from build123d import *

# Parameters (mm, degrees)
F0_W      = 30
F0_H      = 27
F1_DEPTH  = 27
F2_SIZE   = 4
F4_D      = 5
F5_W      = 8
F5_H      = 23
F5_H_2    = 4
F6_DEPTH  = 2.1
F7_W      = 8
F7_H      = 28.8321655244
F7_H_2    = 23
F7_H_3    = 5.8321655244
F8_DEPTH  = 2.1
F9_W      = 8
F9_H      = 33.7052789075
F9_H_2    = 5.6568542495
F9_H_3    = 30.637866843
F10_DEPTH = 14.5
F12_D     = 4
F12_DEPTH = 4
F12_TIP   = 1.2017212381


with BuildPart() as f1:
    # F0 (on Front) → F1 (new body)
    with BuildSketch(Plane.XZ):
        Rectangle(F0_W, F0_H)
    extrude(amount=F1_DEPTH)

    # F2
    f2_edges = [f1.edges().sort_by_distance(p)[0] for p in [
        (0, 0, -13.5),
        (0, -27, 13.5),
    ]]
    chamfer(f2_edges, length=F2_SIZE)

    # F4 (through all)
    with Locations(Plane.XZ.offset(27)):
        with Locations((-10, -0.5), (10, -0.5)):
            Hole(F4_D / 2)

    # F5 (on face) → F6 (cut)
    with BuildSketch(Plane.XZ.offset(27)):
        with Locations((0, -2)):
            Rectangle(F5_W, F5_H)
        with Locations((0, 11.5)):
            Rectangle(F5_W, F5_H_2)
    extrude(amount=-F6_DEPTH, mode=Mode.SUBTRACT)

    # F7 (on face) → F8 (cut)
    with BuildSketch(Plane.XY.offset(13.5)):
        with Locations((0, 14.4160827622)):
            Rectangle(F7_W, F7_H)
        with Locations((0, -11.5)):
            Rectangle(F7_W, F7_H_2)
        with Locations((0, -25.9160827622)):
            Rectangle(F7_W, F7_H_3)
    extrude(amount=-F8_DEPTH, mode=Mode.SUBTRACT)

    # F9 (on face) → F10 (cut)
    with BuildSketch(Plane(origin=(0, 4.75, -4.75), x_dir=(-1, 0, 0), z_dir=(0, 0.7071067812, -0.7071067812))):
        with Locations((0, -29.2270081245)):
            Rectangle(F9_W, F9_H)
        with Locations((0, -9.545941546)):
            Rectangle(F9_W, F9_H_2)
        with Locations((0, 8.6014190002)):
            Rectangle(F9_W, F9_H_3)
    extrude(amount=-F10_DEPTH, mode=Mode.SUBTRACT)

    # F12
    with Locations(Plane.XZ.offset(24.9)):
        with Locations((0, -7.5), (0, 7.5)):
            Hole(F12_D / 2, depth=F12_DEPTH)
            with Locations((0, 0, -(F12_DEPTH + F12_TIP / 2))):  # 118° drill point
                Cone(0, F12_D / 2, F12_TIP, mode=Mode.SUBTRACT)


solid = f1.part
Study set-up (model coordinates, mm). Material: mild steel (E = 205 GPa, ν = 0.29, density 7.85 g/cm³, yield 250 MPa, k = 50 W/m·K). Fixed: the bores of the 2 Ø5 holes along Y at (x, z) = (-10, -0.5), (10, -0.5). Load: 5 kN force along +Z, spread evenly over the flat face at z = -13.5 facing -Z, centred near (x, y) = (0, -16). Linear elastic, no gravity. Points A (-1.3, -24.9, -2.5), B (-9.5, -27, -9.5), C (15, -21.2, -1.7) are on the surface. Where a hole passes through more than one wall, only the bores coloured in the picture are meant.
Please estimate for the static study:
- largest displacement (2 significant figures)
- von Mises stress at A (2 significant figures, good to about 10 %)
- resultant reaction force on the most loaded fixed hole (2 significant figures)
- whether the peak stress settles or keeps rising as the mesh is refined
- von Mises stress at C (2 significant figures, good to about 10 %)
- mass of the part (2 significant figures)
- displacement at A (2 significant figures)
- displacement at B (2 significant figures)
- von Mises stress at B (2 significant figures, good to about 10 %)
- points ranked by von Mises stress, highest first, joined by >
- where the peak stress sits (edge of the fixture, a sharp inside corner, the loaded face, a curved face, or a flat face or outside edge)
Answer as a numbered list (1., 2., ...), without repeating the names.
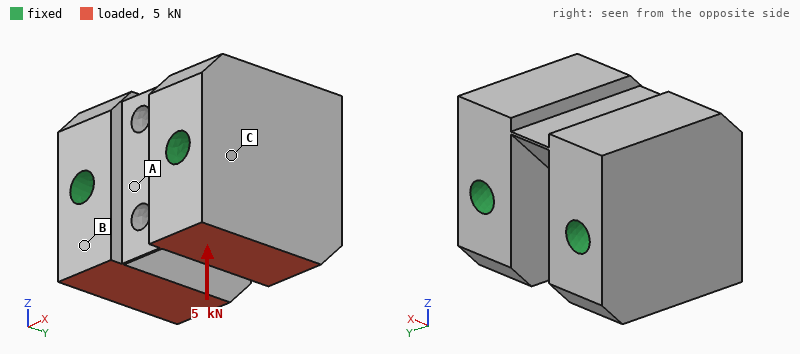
1. 0.72 µm
2. 2.4 MPa
3. 2.5 kN
4. keeps rising
5. 5.6 MPa
6. 130 g
7. 0.21 µm
8. 0.48 µm
9. 11 MPa
10. B > C > A
11. edge of the fixture
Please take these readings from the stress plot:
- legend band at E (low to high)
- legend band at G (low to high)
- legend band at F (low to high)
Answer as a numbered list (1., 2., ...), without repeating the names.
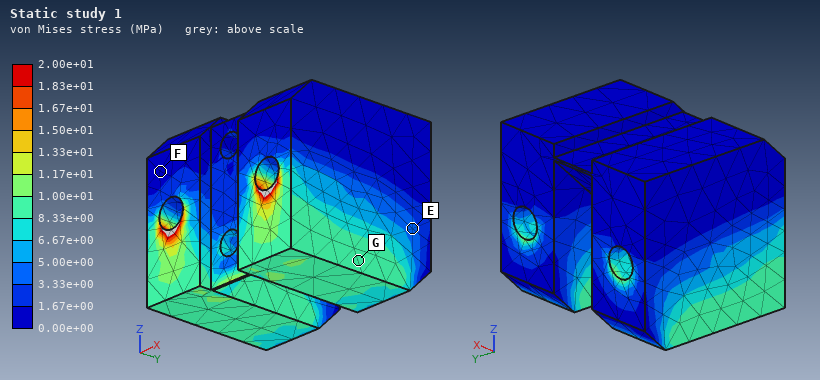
1. 3.33e+00 to 5.00e+00 MPa
2. 8.33e+00 to 1.00e+01 MPa
3. 0.00e+00 to 1.67e+00 MPa
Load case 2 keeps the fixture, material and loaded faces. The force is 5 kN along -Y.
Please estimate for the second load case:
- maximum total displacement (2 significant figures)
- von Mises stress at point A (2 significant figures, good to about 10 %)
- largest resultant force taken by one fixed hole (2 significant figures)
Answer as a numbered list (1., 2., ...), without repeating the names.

1. 2.7 µm
2. 6.1 MPa
3. 2.5 kN
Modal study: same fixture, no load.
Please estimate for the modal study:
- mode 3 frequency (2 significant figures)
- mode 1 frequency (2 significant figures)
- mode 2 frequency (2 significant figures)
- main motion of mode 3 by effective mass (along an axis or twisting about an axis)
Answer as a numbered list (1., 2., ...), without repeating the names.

1. 48 kHz
2. 43 kHz
3. 44 kHz
4. along X
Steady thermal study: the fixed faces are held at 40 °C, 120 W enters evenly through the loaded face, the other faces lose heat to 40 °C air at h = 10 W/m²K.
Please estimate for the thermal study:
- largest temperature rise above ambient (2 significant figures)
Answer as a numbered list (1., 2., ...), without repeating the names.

1. 51 K
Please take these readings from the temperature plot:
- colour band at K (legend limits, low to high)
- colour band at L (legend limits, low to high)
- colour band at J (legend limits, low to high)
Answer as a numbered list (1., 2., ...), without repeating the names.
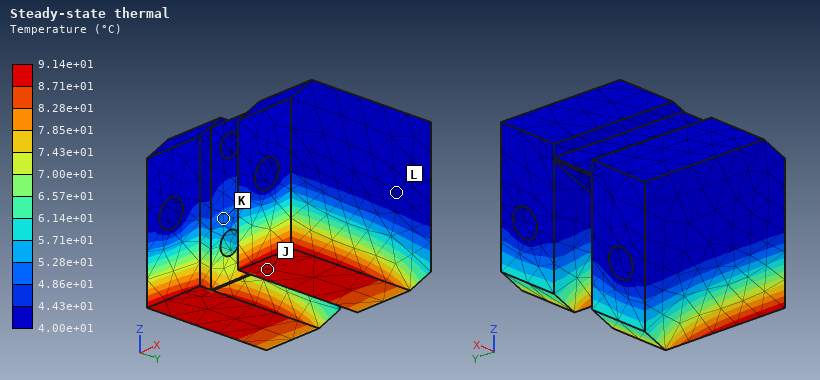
1. 4.86e+01 to 5.28e+01 °C
2. 4.00e+01 to 4.43e+01 °C
3. 8.71e+01 to 9.14e+01 °C
